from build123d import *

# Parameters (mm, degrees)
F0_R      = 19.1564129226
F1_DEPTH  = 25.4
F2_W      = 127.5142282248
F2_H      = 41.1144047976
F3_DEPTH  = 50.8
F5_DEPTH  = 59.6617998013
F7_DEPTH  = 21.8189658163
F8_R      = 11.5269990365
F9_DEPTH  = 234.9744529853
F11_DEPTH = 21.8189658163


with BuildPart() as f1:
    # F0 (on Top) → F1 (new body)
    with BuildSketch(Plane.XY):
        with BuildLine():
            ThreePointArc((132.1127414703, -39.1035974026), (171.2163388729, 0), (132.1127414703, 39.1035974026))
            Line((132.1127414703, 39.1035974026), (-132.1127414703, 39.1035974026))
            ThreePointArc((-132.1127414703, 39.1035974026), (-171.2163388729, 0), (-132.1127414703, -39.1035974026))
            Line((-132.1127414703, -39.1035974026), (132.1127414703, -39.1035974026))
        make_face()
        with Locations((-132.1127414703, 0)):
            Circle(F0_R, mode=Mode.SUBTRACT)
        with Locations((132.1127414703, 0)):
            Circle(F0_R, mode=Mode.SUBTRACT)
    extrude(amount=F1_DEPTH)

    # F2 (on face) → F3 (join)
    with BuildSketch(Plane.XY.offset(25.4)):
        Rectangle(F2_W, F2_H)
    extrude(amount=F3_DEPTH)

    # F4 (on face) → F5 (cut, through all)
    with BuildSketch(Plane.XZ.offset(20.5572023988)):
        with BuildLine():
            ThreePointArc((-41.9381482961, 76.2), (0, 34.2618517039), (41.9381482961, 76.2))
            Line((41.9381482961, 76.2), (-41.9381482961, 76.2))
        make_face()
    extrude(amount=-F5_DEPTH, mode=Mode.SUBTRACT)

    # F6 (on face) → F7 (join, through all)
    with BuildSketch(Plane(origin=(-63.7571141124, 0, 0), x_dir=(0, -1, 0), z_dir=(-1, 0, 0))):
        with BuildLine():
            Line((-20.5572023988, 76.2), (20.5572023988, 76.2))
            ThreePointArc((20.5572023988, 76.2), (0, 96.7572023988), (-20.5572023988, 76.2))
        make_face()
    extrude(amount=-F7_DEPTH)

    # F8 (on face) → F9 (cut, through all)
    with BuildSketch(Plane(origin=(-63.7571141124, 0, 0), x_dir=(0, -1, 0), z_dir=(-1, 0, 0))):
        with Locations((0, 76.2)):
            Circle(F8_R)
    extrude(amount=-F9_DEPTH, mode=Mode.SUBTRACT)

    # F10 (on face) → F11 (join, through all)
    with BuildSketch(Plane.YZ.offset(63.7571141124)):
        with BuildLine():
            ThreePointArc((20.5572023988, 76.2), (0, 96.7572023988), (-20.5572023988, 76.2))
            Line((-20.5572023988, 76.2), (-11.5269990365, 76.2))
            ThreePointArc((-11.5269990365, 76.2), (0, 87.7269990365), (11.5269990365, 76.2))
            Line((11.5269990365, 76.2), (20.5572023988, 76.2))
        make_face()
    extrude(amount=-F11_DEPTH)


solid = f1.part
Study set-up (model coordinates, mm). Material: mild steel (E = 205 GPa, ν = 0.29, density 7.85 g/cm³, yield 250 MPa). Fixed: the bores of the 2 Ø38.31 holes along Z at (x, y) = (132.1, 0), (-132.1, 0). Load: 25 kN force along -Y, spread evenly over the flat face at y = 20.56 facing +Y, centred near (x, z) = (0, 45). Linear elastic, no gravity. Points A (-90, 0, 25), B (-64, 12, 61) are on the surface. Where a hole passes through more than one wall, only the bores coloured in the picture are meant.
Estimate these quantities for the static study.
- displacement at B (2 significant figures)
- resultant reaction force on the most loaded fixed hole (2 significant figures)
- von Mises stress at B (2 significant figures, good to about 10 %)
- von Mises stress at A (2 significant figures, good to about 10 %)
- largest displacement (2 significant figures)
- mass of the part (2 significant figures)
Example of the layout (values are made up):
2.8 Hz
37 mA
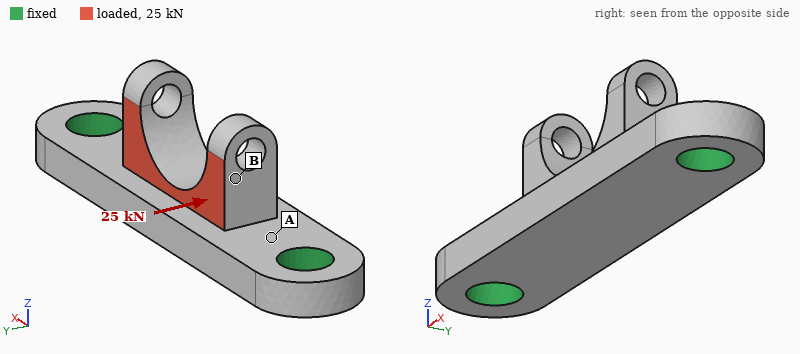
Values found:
58 µm
13 kN
10 MPa
56 MPa
92 µm
5.9 kg
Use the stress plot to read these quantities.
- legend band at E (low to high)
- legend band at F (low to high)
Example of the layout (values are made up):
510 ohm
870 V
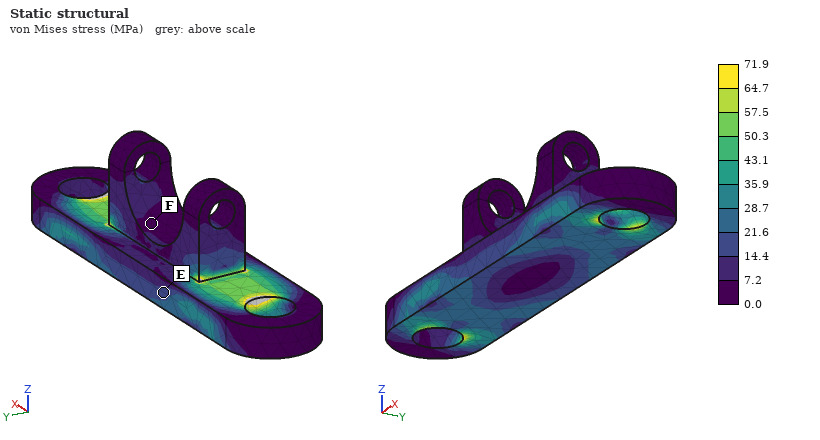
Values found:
14.4 to 21.6 MPa
0.0 to 7.2 MPa
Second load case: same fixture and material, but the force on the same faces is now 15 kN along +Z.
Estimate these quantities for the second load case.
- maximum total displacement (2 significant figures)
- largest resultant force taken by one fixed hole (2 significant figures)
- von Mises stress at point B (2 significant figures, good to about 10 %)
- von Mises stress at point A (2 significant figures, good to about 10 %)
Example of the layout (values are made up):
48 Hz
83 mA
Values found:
42 µm
8.1 kN
5.2 MPa
18 MPa
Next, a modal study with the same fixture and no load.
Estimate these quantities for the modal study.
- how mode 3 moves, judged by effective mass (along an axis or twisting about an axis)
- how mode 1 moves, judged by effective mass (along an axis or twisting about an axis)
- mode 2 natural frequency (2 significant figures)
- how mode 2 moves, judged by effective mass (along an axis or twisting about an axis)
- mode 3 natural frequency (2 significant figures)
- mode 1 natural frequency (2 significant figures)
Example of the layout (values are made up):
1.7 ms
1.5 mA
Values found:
along Y
along Z
2400 Hz
along Y
3900 Hz
2100 Hz
